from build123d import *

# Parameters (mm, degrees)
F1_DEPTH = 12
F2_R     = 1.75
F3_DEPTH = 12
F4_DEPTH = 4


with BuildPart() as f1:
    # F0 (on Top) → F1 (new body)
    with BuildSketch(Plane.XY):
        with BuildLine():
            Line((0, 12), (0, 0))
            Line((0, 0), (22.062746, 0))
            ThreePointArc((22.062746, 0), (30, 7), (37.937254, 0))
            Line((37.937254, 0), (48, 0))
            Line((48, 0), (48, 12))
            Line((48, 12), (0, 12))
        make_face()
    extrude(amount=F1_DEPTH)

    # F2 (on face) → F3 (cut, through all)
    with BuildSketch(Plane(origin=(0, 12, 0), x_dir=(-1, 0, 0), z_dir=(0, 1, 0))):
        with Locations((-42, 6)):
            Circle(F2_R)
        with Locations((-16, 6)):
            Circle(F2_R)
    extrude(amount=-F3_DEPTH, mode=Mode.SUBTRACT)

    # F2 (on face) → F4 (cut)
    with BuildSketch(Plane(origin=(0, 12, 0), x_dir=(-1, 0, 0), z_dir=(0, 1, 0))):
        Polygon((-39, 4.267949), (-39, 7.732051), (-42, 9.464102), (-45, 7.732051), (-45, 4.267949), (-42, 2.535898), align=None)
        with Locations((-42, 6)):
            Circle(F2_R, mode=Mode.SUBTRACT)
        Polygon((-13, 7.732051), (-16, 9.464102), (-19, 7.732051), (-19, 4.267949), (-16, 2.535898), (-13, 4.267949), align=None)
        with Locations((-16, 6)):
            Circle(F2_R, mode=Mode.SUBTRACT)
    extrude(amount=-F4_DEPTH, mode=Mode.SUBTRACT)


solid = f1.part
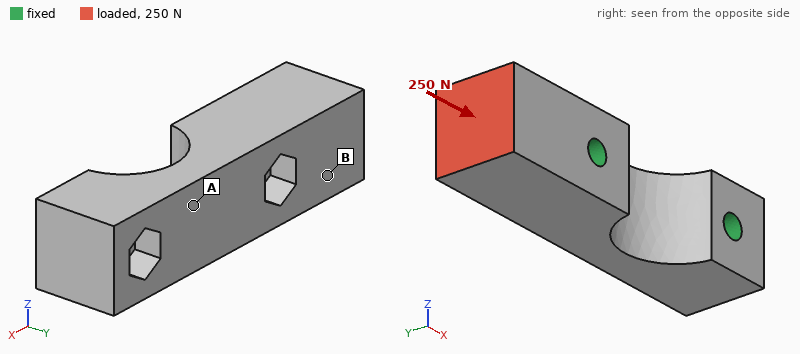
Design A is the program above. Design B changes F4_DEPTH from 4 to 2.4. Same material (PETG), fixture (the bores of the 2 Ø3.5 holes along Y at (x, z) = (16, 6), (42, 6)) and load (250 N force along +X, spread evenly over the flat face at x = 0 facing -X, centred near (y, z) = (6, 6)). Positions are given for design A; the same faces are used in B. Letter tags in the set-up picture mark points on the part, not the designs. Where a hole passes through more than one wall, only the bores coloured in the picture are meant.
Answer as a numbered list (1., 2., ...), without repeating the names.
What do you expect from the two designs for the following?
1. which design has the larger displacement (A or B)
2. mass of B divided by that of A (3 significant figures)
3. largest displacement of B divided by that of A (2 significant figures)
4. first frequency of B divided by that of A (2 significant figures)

1. A
2. 1.01
3. 0.68
4. 1.1
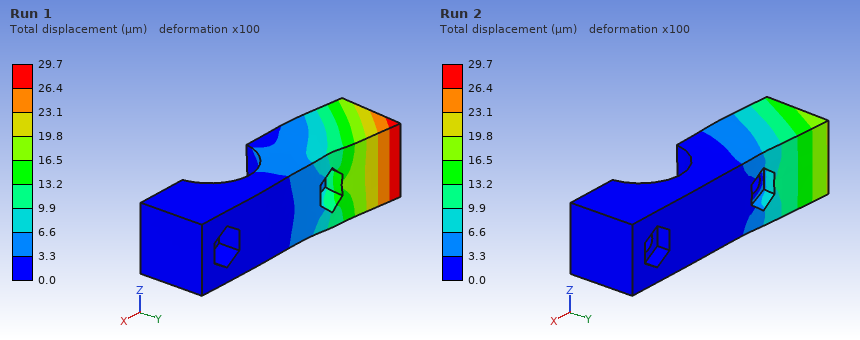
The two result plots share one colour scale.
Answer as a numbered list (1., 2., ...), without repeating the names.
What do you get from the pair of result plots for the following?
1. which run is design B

1. Run 2
